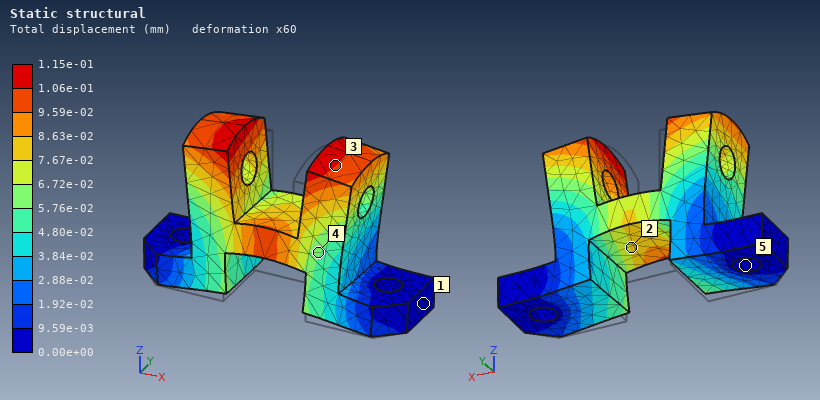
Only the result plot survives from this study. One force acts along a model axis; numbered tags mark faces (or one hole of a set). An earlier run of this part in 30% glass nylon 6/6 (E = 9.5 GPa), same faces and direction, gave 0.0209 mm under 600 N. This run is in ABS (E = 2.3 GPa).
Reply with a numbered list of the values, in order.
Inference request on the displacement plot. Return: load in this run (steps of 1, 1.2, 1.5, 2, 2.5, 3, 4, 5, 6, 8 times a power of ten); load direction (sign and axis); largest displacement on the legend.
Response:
1. 800 N
2. +Z
3. 1.15e-01 mm
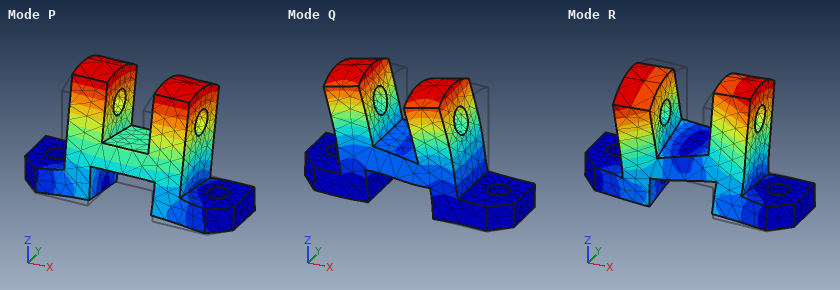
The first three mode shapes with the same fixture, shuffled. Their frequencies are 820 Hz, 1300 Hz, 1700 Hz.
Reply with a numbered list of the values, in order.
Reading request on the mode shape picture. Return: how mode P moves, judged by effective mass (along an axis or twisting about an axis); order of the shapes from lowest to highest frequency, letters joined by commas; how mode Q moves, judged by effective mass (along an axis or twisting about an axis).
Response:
1. along Y
2. P, R, Q
3. along X
